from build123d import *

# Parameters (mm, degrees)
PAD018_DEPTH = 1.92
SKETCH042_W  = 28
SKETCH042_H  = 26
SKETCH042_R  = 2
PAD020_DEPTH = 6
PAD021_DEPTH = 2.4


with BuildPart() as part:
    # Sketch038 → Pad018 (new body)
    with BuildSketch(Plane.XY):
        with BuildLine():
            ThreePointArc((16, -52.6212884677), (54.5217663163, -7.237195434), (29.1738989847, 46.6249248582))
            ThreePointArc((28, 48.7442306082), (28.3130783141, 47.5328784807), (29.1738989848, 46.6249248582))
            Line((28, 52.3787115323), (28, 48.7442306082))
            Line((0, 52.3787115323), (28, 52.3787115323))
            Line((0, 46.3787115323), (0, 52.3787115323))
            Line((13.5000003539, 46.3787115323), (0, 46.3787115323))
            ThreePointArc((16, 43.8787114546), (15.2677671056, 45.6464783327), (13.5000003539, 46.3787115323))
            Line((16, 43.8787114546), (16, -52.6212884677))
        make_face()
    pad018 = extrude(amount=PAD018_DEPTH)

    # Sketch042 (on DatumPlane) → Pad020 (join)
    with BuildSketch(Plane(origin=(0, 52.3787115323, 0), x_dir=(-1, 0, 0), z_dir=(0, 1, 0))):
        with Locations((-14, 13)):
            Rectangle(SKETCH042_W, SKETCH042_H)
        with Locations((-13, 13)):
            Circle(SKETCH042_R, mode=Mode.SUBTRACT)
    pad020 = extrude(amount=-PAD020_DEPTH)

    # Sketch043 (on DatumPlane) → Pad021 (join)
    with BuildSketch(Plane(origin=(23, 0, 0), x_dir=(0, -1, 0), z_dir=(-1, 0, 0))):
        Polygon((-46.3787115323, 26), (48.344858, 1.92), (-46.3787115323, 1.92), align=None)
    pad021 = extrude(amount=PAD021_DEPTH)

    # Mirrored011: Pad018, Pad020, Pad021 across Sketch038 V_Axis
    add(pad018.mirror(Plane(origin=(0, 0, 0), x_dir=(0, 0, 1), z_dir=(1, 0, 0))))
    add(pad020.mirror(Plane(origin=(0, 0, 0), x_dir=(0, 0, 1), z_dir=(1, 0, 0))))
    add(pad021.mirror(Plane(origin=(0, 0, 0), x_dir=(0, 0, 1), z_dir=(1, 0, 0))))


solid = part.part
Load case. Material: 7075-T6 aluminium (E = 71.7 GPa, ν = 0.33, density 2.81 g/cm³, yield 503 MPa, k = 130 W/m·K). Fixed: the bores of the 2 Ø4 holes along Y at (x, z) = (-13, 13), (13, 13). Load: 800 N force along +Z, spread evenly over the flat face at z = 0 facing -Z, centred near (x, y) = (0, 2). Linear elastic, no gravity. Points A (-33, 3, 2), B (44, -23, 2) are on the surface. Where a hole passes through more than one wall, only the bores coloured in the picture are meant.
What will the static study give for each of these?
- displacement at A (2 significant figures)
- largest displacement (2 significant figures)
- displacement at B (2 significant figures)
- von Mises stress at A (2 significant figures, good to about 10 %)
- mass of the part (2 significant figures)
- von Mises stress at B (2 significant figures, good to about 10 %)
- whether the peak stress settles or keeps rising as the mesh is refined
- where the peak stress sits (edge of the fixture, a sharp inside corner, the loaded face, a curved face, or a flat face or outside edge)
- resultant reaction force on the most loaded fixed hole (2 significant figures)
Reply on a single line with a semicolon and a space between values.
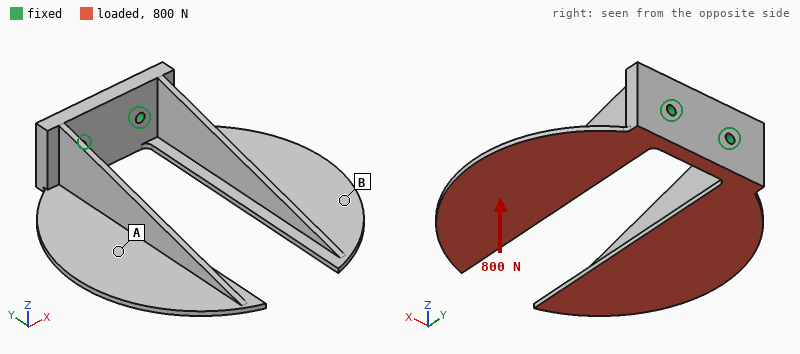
0.59 mm; 1.6 mm; 1.3 mm; 47 MPa; 72 g; 16 MPa; keeps rising; edge of the fixture; 400 N
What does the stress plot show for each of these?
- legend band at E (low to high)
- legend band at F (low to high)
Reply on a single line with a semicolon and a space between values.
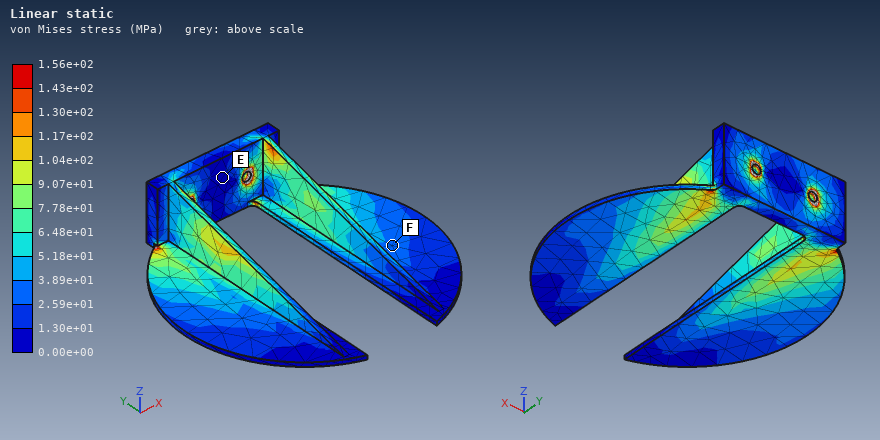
0.00e+00 to 1.30e+01 MPa; 2.59e+01 to 3.89e+01 MPa
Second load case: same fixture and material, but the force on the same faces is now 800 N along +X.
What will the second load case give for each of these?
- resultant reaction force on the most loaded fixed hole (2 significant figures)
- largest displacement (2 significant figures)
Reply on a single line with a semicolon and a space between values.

760 N; 1.5 mm
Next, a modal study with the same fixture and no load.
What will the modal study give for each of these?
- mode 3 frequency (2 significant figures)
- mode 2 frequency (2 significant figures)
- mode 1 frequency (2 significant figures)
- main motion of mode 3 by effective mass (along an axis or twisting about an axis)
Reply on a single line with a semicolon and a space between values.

790 Hz; 710 Hz; 690 Hz; along Z
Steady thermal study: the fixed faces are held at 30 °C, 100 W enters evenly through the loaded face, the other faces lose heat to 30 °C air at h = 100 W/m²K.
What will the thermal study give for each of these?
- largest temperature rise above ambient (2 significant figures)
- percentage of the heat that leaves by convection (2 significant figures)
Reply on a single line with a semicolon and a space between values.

79 K; 64 %
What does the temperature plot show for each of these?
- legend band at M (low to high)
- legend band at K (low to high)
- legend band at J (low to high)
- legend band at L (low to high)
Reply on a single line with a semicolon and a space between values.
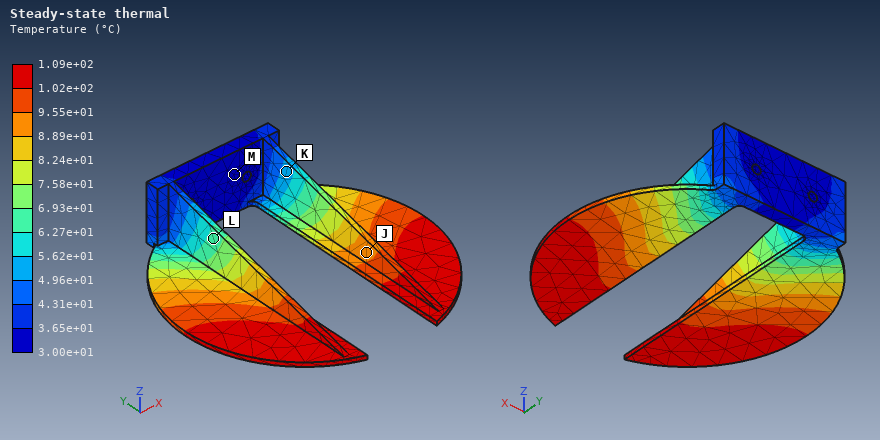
3.00e+01 to 3.65e+01 °C; 4.96e+01 to 5.62e+01 °C; 8.89e+01 to 9.55e+01 °C; 6.27e+01 to 6.93e+01 °C
